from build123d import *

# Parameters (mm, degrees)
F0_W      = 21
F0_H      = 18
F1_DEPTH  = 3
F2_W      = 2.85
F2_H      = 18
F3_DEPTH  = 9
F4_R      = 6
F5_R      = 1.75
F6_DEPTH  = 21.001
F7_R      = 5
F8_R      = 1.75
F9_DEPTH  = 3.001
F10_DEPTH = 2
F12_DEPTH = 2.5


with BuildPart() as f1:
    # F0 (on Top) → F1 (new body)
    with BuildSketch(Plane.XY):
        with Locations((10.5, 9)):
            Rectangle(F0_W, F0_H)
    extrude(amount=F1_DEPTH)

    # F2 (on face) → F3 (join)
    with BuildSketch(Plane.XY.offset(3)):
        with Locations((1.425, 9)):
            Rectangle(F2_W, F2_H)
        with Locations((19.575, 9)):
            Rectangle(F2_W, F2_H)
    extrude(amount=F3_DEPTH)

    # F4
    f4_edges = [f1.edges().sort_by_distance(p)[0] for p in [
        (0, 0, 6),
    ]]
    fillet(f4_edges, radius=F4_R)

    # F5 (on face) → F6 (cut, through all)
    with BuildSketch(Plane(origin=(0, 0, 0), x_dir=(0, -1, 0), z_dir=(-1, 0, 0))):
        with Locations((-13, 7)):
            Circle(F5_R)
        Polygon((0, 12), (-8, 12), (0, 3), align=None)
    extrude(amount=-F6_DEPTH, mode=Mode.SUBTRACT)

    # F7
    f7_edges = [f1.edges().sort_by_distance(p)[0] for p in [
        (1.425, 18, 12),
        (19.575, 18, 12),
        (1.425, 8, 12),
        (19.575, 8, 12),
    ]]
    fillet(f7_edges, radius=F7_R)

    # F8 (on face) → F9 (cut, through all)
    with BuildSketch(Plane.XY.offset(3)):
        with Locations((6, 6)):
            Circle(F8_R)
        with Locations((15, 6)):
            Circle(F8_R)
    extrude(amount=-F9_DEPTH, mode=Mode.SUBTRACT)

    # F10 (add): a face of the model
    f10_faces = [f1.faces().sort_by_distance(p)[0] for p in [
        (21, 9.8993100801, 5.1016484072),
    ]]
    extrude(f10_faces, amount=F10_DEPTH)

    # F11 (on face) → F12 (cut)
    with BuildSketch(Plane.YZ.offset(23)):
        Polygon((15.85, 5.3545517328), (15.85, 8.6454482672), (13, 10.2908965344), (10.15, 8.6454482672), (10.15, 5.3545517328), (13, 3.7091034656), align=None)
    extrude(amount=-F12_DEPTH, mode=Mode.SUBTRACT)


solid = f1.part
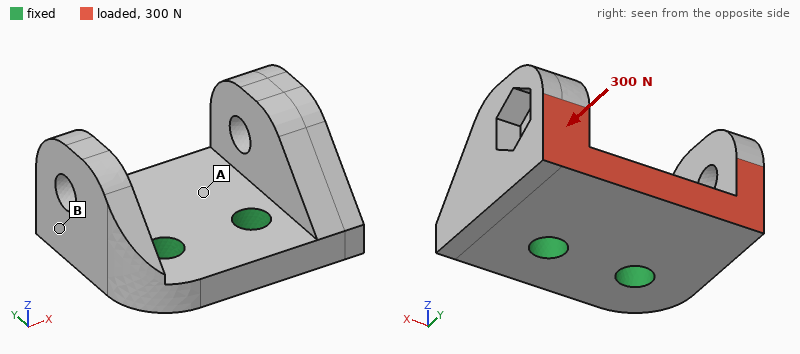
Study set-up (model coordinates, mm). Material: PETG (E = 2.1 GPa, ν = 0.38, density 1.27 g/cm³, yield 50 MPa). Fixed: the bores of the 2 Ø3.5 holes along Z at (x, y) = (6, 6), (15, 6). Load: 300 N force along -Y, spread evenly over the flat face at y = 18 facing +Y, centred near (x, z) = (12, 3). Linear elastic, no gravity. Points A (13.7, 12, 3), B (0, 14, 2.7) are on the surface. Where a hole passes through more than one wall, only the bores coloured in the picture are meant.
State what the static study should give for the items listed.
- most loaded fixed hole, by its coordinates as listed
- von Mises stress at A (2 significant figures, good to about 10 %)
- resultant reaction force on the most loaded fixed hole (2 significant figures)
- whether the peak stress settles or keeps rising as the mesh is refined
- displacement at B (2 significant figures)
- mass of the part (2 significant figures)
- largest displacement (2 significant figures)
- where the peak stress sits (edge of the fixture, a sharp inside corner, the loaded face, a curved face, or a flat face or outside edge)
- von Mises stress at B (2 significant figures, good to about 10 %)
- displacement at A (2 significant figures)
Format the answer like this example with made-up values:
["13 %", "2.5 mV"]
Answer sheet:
["(15, 6)", "5.7 MPa", "190 N", "keeps rising", "0.037 mm", "2.5 g", "0.11 mm", "edge of the fixture", "2.9 MPa", "0.028 mm"]
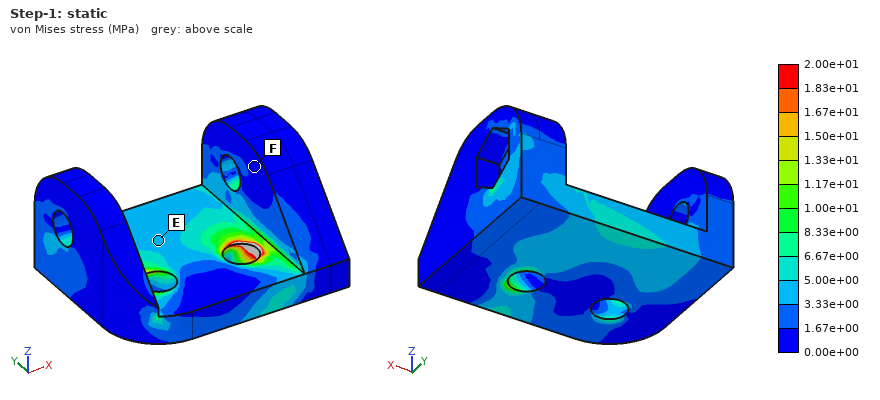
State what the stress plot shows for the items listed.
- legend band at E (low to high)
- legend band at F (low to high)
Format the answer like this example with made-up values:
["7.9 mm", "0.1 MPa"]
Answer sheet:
["3.33e+00 to 5.00e+00 MPa", "0.00e+00 to 1.67e+00 MPa"]
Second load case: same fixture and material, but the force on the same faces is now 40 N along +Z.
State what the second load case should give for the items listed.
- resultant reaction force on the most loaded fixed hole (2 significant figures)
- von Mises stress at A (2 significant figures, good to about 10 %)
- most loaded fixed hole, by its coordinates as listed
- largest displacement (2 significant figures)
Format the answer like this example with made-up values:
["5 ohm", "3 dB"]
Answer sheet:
["24 N", "3.4 MPa", "(15, 6)", "0.13 mm"]
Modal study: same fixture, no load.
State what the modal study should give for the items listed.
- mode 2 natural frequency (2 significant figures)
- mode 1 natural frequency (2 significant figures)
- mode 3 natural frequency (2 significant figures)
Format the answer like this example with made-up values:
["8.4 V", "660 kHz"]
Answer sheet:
["3700 Hz", "3100 Hz", "4100 Hz"]
